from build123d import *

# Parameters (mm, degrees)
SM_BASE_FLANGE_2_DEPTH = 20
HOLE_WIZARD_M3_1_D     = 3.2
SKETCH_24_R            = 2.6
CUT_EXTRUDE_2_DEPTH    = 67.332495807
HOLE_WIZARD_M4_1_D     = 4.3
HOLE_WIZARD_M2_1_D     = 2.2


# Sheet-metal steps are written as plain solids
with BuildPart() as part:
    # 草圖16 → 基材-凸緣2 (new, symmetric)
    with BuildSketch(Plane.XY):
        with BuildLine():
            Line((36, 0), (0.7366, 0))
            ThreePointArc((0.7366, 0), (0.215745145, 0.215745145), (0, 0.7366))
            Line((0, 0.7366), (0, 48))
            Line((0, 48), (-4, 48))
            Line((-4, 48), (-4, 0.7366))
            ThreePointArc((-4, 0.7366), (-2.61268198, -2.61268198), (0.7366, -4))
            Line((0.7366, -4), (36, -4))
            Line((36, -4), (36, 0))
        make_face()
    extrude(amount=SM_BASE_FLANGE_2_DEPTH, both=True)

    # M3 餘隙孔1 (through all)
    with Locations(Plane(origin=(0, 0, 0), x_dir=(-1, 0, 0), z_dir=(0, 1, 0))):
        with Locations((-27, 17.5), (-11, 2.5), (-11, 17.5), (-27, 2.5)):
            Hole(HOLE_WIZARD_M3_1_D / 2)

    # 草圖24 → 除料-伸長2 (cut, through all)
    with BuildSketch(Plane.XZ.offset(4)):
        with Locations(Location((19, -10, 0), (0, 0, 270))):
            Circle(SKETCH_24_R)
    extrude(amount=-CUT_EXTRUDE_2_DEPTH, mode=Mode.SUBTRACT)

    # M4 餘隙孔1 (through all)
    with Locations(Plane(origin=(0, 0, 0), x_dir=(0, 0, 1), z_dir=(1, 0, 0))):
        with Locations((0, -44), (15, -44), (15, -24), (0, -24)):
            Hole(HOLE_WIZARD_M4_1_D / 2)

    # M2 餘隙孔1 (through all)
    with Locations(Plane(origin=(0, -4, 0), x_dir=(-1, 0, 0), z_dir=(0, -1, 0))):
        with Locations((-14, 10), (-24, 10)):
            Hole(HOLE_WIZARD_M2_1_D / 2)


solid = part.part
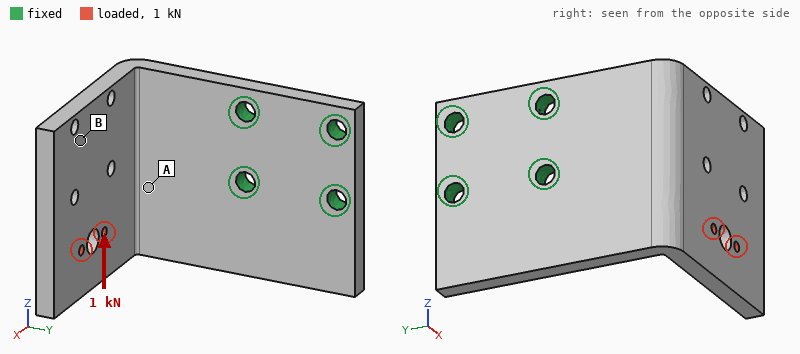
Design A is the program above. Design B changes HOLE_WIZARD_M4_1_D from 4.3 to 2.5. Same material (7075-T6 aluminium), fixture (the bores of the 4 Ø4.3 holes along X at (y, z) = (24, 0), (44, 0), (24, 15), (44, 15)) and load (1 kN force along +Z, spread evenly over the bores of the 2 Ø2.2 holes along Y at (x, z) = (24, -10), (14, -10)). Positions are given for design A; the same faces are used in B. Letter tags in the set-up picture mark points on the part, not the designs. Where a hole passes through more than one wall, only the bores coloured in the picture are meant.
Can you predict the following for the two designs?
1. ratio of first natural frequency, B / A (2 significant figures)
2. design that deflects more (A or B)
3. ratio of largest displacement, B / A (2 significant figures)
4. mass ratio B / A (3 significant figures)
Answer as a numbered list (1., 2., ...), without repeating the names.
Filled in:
1. 0.96
2. B
3. 1.1
4. 1.01
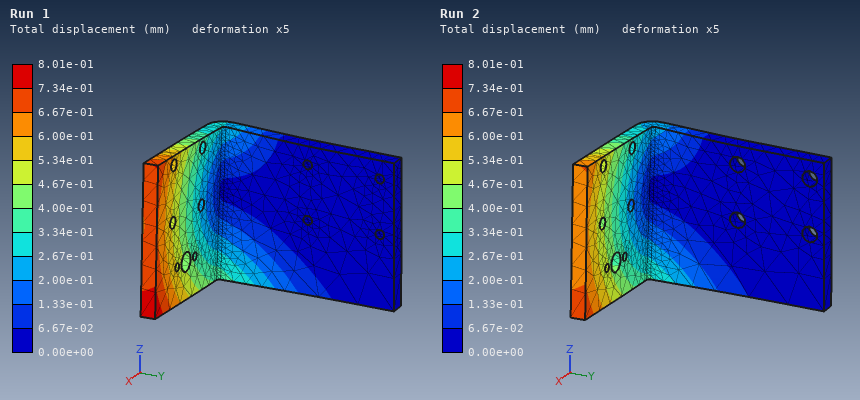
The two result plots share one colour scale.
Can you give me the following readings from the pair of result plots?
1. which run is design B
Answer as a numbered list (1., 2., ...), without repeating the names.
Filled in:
1. Run 1
